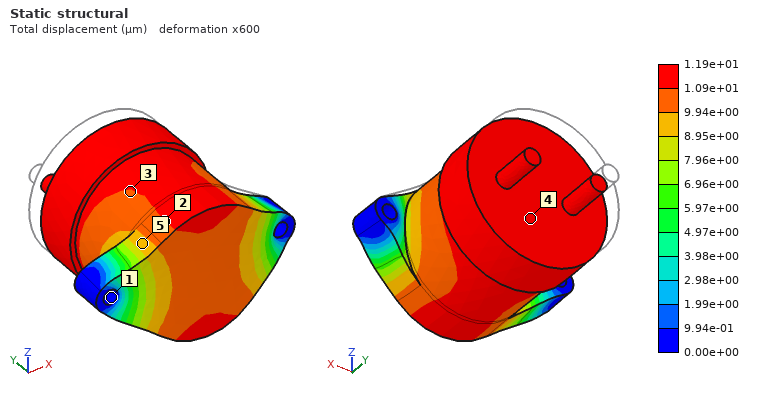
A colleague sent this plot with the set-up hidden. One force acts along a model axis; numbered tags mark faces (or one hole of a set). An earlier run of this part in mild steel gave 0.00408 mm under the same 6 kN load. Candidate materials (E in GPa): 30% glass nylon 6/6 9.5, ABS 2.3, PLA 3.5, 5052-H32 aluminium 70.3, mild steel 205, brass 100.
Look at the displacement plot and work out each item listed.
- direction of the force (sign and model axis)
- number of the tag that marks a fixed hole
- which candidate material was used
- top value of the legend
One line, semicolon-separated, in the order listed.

-Y; 1; 5052-H32 aluminium; 1.19e+01 µm
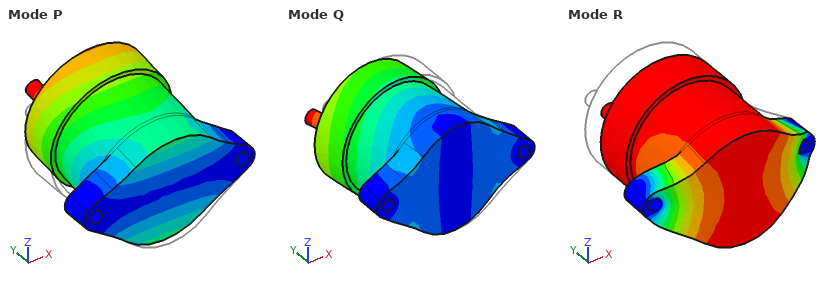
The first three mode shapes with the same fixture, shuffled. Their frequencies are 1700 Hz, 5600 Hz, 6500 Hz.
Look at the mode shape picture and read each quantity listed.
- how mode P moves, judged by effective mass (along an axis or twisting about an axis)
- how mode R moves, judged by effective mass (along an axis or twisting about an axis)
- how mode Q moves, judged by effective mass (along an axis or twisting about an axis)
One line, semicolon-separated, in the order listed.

along Z; along Y; along X
